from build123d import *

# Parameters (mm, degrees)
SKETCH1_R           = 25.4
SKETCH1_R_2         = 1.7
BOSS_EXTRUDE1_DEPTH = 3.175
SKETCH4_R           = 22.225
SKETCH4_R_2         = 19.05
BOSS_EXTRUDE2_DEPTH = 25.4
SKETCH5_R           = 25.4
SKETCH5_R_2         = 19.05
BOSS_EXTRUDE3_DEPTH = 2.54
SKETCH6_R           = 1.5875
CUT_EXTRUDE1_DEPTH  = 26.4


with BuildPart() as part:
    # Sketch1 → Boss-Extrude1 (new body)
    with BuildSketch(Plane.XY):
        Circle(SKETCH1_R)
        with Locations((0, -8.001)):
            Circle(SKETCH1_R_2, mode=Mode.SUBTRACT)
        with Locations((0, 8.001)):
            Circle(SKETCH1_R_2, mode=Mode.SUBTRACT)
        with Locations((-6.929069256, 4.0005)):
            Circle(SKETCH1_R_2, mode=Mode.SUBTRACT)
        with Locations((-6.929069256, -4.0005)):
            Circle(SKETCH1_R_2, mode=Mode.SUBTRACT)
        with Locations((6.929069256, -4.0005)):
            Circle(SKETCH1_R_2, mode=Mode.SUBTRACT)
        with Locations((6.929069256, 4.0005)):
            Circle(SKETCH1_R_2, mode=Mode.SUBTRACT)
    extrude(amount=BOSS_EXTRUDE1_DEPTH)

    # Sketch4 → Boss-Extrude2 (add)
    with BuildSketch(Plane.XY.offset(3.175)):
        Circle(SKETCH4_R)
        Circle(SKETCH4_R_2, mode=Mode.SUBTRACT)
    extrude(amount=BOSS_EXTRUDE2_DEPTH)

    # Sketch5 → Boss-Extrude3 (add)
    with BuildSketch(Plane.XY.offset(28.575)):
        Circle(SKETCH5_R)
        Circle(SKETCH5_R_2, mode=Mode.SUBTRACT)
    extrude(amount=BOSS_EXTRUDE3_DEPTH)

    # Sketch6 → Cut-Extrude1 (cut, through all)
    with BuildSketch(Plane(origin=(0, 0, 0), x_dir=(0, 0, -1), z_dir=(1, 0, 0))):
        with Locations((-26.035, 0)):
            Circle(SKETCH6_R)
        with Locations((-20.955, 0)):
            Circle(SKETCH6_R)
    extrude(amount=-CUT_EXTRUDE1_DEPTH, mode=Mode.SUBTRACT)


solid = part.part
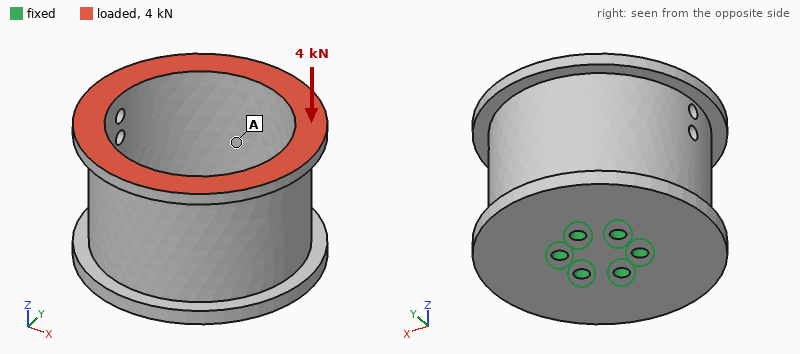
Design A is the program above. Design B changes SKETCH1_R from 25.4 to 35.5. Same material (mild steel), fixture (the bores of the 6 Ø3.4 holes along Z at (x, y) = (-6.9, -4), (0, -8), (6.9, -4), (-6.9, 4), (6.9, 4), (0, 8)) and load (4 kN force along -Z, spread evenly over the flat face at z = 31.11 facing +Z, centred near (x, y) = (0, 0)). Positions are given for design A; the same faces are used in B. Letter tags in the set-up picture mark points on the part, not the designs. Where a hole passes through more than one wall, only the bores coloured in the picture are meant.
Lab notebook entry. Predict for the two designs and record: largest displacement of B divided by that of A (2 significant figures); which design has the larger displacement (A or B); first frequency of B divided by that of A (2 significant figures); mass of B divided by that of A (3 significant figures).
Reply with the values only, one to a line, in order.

1.3
B
0.84
1.32
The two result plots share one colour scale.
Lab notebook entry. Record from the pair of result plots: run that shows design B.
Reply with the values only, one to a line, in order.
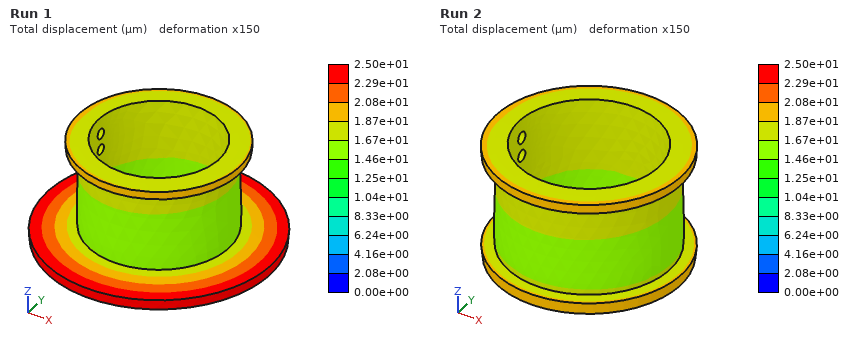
Run 1
